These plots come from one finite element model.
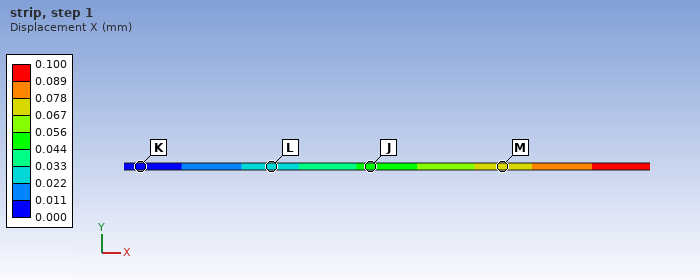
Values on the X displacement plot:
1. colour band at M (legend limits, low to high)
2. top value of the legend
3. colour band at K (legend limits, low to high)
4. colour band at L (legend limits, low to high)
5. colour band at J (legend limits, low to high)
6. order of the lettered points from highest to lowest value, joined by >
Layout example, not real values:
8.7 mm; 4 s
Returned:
0.067 to 0.078 mm; 0.100 mm; 0.000 to 0.011 mm; 0.022 to 0.033 mm; 0.044 to 0.056 mm; M > J > L > K
